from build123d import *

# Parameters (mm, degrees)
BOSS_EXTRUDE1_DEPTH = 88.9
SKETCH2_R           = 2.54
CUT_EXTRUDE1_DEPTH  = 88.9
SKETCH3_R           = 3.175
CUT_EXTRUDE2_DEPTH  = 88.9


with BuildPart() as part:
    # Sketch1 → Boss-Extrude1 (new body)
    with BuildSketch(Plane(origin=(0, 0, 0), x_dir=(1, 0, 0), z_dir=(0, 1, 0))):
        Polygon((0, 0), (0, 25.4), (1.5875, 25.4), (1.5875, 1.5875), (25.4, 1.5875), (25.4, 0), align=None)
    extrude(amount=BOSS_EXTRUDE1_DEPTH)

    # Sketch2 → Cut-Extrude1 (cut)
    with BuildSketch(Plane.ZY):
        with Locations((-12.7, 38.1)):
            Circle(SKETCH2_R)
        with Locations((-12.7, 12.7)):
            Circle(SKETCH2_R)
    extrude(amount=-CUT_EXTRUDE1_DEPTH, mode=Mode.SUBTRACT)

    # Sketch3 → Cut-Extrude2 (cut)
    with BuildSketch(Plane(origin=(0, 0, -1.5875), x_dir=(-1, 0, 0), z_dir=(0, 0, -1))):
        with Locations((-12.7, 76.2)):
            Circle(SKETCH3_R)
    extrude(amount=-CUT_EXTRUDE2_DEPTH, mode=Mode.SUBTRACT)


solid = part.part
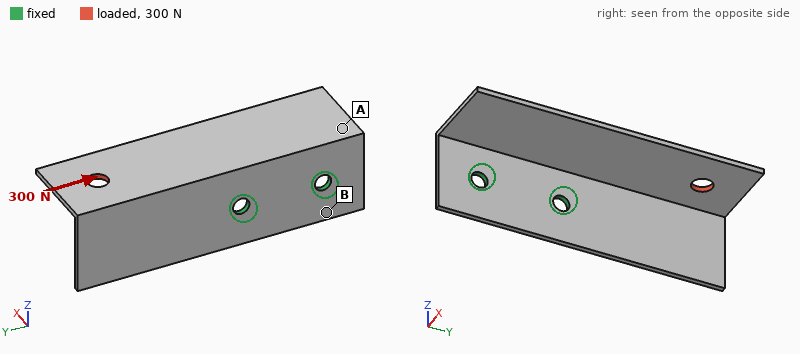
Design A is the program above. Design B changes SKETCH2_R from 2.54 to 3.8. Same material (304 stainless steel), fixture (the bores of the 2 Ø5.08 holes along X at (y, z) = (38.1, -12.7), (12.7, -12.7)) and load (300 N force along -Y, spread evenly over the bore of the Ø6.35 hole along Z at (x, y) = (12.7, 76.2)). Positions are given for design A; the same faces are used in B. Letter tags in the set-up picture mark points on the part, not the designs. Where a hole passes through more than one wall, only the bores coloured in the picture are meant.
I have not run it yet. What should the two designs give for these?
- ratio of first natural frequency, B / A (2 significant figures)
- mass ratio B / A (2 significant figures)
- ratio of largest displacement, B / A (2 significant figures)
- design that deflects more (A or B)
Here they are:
1.1
0.99
0.73
A
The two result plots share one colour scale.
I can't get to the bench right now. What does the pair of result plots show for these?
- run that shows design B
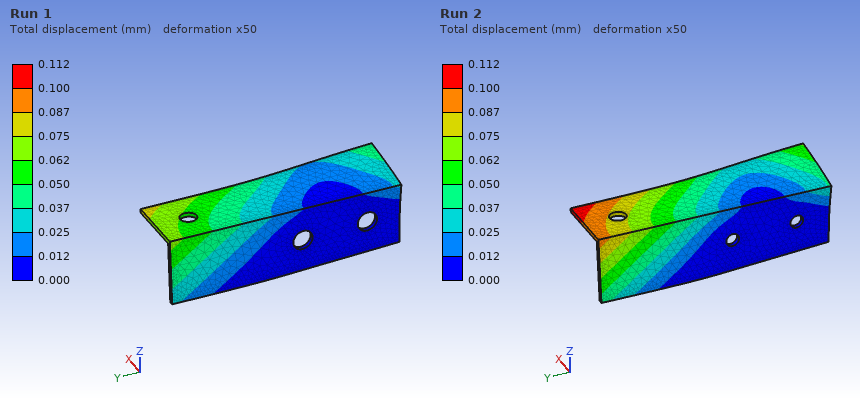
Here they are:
Run 1
